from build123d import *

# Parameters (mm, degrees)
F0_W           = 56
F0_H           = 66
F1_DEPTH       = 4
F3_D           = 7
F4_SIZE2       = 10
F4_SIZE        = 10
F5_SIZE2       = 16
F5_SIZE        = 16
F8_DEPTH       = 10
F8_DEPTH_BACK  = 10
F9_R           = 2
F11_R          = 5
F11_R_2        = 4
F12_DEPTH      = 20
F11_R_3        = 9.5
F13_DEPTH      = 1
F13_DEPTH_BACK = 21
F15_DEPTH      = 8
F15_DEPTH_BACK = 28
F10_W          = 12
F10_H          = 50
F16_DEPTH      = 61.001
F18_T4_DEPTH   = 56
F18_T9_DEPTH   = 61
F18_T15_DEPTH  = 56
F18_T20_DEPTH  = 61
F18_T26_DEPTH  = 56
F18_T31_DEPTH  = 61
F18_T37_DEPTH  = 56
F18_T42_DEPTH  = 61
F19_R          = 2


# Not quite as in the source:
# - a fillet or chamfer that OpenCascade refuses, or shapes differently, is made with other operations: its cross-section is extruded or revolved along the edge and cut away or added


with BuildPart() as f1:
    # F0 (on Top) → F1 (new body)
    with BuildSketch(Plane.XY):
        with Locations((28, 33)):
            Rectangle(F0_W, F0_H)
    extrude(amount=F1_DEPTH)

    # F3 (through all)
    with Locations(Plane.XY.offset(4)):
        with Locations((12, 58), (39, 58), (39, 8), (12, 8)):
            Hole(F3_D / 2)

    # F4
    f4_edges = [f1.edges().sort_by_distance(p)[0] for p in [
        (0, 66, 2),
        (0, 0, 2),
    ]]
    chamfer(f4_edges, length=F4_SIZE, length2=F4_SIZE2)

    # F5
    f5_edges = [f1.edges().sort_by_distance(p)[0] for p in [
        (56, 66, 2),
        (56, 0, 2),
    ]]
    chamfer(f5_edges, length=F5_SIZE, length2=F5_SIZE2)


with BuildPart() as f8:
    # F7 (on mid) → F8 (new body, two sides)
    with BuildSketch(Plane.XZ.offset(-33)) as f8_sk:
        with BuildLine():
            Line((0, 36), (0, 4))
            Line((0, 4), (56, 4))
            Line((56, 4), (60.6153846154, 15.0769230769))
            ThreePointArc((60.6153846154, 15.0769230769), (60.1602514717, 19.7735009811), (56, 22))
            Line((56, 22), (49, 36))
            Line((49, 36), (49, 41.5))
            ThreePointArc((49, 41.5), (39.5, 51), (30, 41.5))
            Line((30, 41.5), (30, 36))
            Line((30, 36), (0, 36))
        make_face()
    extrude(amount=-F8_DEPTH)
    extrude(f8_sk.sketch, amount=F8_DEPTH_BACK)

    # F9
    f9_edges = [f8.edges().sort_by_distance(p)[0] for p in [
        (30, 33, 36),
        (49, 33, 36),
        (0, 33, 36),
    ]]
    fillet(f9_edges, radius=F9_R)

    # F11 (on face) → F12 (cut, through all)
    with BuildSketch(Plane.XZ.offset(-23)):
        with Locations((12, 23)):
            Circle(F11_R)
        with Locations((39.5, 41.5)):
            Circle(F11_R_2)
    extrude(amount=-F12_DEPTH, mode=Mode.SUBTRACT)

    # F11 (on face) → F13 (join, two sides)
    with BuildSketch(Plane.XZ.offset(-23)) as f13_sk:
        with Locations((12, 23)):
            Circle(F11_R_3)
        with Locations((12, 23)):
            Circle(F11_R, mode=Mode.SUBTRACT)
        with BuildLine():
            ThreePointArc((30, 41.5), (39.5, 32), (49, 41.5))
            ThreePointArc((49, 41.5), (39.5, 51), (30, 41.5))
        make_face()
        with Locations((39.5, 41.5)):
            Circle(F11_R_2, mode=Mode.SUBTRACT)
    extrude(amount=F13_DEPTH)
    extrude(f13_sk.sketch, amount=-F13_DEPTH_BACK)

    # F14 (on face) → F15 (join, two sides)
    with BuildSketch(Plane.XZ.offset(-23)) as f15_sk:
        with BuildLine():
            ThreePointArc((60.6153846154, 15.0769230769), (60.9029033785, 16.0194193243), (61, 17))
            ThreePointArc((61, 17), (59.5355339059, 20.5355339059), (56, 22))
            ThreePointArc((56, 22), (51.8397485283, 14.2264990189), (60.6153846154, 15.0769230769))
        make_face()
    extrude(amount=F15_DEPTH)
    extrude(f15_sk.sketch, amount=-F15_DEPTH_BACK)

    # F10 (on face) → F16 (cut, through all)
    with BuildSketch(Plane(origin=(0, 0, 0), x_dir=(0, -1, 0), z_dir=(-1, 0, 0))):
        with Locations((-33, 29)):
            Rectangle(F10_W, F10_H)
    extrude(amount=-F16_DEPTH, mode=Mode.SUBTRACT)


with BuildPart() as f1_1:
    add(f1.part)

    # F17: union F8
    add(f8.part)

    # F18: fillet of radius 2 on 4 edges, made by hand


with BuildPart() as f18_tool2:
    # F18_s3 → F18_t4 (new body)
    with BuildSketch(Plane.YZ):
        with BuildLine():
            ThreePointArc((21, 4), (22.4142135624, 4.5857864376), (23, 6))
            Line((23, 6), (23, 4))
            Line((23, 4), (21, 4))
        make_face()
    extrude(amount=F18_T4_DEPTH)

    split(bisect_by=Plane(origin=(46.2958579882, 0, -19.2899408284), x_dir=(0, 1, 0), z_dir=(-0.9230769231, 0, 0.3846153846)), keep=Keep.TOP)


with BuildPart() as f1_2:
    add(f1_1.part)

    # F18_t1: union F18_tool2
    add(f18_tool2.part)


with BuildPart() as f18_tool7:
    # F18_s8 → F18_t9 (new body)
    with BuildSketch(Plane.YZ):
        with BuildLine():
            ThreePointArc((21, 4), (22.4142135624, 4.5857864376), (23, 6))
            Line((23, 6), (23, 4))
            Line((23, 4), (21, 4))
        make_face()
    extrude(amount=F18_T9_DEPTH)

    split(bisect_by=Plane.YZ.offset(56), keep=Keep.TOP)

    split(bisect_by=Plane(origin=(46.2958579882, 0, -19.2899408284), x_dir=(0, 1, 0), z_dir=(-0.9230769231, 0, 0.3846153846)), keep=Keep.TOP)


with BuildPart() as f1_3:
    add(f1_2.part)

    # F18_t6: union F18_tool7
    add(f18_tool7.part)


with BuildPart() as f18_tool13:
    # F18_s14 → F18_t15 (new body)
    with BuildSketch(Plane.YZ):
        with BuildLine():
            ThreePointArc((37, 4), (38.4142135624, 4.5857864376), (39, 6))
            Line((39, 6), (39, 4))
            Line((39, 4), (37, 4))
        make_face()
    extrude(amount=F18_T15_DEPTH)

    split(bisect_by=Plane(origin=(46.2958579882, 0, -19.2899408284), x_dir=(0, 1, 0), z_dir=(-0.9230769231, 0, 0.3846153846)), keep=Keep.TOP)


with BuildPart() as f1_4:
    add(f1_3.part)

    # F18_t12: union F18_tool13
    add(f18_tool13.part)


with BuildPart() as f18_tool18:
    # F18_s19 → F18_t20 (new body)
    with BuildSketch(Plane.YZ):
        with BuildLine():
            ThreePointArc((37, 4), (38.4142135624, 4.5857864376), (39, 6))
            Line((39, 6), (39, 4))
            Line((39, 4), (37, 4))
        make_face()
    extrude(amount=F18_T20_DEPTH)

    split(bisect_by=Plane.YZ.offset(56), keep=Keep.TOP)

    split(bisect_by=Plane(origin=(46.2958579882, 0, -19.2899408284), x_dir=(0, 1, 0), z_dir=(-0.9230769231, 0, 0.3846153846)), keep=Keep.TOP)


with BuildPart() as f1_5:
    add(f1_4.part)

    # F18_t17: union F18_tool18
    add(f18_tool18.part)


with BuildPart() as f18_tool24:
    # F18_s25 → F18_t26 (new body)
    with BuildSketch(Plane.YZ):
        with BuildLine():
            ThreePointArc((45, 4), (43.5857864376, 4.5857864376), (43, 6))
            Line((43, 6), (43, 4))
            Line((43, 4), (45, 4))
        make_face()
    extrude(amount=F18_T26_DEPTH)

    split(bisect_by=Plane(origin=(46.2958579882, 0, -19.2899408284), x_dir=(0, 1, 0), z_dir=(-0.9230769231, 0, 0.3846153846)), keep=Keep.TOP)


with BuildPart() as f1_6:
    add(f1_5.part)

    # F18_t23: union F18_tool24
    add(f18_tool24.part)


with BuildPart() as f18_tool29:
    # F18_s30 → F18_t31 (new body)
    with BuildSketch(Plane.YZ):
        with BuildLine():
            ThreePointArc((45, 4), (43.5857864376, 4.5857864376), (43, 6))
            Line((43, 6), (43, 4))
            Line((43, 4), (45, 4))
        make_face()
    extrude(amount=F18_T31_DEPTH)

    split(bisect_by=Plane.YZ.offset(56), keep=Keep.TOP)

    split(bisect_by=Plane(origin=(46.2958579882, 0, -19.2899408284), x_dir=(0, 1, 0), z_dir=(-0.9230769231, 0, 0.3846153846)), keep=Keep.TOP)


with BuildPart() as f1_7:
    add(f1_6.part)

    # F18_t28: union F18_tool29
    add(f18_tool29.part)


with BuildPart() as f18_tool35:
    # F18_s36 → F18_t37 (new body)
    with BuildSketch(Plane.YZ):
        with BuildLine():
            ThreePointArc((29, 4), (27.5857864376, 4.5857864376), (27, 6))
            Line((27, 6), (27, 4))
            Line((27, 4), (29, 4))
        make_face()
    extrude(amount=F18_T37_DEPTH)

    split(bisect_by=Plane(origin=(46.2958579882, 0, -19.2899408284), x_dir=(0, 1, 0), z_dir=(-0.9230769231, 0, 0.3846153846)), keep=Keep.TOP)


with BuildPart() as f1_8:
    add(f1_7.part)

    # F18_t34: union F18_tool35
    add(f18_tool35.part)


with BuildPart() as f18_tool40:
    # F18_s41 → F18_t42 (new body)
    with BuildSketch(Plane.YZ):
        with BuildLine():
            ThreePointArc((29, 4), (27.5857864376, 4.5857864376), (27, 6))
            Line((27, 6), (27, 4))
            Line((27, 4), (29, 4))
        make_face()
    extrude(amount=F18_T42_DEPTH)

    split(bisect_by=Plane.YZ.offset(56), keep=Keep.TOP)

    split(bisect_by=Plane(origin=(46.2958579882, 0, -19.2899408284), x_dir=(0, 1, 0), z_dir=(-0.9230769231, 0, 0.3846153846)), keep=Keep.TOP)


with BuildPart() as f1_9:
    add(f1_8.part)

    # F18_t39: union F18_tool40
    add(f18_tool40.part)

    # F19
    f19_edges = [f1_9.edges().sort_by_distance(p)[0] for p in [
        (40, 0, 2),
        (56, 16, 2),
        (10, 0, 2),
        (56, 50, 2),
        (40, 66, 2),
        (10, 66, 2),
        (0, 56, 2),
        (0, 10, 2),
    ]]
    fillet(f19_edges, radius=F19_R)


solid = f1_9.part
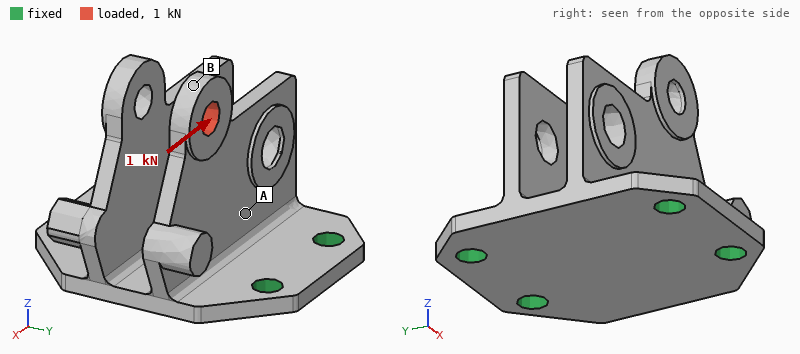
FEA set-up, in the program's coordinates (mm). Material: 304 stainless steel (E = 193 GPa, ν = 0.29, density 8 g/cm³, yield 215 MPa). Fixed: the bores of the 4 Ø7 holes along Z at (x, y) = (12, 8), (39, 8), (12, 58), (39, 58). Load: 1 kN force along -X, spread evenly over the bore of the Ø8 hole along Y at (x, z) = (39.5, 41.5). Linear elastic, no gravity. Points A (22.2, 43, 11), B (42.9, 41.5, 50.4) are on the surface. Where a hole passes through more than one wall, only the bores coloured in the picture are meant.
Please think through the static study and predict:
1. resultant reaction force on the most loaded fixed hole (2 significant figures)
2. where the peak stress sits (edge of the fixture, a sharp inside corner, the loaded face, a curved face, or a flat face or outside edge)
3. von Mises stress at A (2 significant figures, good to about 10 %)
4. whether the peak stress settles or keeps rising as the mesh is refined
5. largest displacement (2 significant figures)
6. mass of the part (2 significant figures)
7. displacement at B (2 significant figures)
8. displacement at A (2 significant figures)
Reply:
910 N
edge of the fixture
23 MPa
keeps rising
58 µm
240 g
57 µm
10 µm
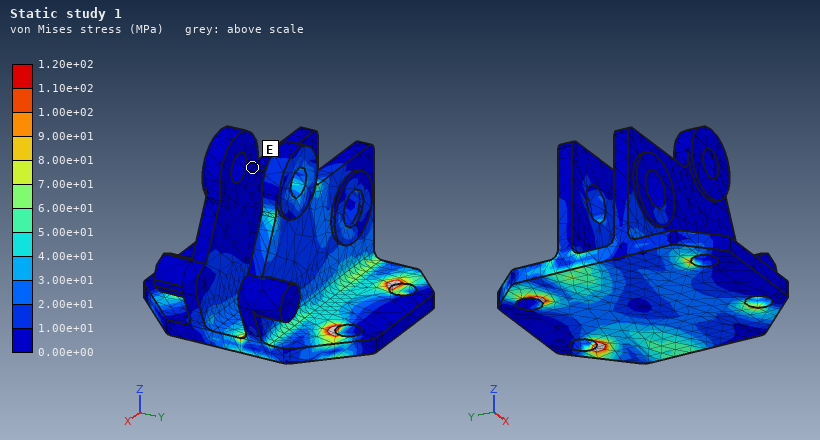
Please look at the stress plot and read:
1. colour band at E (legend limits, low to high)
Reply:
0.00e+00 to 1.00e+01 MPa
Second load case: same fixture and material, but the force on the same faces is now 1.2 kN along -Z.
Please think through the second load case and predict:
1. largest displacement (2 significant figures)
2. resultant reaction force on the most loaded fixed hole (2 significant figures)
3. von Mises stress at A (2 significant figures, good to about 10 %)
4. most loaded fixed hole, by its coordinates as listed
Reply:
31 µm
800 N
6.6 MPa
(39, 58)
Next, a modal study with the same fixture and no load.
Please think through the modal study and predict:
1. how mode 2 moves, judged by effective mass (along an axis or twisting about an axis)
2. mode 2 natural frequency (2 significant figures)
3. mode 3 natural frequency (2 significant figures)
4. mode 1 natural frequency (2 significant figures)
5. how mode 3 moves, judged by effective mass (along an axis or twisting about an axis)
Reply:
along Y
2100 Hz
3000 Hz
1800 Hz
along X
